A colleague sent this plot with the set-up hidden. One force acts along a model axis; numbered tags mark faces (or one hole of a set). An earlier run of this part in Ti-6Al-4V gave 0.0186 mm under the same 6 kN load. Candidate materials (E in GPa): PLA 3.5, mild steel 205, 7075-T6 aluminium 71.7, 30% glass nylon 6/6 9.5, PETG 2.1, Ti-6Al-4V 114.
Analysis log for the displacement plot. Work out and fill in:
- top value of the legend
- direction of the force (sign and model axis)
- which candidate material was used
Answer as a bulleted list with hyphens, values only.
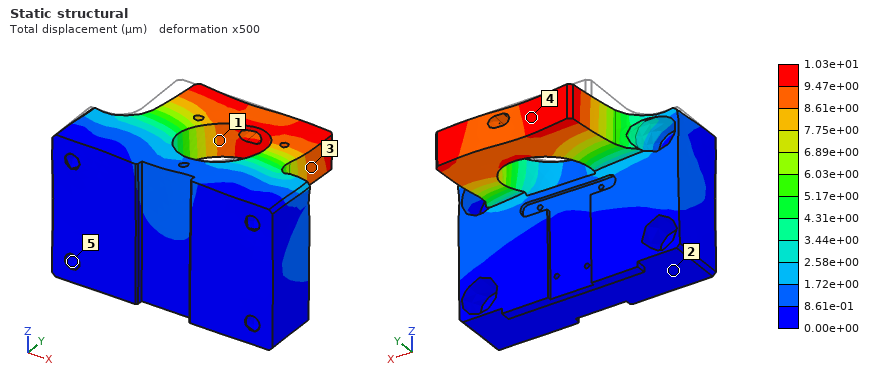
- 1.03e+01 µm
- +X
- mild steel
